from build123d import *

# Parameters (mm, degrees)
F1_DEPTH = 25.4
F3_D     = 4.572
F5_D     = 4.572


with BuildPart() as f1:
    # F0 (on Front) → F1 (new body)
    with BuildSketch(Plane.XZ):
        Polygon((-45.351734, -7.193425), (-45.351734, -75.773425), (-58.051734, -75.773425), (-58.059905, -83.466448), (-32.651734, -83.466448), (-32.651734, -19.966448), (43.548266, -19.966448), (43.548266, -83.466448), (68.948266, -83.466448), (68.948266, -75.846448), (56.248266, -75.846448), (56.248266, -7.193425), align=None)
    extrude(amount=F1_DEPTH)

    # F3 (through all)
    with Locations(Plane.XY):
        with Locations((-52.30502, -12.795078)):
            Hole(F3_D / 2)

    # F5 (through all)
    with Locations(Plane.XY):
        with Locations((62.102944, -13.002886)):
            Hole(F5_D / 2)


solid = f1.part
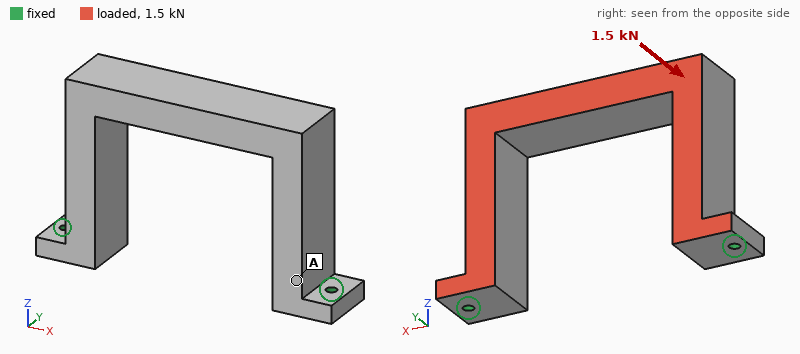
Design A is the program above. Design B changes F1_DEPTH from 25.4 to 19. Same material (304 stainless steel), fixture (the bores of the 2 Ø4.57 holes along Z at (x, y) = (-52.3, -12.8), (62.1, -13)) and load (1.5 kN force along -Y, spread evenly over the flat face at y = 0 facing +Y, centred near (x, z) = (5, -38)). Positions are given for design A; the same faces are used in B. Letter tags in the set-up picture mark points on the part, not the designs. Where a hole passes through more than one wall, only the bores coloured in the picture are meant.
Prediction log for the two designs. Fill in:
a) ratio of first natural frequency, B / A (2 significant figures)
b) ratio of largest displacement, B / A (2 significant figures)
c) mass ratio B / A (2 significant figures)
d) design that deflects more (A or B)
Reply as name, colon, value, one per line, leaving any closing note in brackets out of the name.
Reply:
ratio of first natural frequency, B / A: 0.95
ratio of largest displacement, B / A: 1.5
mass ratio B / A: 0.75
design that deflects more: B
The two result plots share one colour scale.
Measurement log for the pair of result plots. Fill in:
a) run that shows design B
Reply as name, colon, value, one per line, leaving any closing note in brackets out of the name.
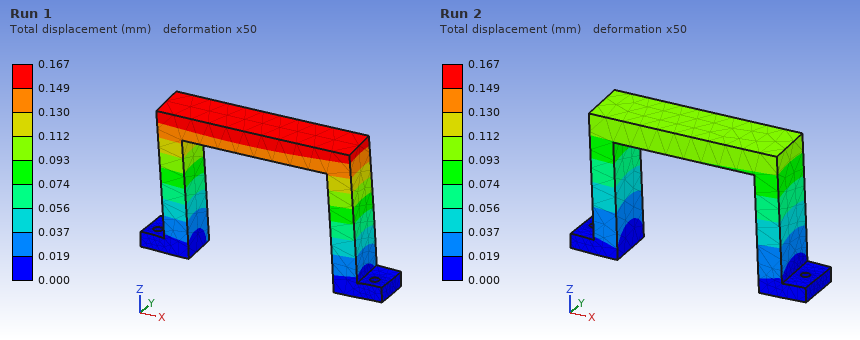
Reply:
run that shows design B: Run 1
